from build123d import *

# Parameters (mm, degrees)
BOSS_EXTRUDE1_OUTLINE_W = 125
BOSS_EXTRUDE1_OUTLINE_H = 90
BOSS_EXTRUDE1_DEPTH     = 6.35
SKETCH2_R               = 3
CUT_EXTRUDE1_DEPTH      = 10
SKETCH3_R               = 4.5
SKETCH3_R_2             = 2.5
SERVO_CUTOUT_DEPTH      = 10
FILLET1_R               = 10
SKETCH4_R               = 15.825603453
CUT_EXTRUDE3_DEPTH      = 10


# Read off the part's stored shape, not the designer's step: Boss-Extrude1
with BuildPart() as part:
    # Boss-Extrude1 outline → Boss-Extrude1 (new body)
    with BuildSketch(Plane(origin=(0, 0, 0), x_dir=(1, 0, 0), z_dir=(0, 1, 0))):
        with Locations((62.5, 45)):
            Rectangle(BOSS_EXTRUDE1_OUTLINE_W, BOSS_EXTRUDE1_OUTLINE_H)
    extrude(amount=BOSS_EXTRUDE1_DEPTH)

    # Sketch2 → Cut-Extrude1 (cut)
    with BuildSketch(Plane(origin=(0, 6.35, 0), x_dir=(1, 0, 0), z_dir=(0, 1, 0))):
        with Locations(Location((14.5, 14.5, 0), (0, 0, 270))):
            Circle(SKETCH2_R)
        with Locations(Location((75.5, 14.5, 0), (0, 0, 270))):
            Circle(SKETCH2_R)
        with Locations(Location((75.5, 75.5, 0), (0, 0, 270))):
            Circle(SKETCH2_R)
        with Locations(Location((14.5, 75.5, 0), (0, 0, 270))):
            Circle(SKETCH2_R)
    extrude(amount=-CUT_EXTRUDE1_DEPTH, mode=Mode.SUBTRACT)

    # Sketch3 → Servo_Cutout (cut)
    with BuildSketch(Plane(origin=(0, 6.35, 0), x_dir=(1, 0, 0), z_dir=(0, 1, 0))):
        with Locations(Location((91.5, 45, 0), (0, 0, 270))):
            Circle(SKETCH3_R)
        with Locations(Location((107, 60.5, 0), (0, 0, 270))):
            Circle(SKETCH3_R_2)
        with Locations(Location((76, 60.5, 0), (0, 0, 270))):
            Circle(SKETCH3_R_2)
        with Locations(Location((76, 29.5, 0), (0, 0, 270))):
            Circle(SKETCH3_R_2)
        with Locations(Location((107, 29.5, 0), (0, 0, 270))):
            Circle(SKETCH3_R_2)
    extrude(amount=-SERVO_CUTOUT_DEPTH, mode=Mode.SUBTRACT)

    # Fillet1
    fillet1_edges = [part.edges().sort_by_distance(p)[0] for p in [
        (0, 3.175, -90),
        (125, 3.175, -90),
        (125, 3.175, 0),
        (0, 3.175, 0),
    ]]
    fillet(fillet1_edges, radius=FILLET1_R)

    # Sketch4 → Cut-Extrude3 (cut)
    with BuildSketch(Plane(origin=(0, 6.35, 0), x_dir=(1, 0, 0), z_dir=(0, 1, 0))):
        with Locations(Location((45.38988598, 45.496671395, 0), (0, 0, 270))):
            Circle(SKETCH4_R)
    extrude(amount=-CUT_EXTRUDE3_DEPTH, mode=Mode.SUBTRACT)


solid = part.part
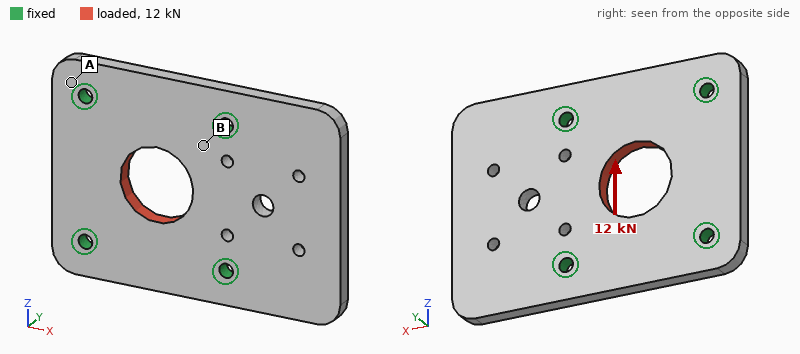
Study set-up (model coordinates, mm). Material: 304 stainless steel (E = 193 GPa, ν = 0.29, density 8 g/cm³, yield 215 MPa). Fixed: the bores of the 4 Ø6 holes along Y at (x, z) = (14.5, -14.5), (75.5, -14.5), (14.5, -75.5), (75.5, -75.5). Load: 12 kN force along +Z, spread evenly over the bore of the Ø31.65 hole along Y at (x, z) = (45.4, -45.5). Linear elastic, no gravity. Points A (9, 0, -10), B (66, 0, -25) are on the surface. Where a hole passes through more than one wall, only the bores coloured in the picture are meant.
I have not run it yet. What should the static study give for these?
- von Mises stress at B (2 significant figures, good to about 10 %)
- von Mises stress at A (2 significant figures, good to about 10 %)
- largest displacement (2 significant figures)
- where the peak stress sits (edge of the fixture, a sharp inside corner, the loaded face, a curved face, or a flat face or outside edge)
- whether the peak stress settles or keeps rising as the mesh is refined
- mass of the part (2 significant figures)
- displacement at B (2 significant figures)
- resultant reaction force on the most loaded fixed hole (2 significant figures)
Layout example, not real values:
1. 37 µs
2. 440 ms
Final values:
1. 21 MPa
2. 9.8 MPa
3. 5.2 µm
4. edge of the fixture
5. keeps rising
6. 510 g
7. 2.3 µm
8. 3.2 kN
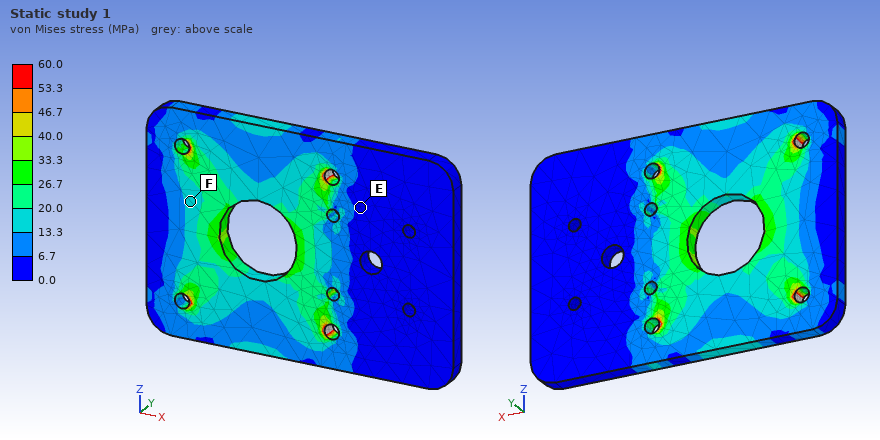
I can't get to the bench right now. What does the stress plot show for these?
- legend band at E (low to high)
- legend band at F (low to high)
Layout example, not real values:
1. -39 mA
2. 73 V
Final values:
1. 0.0 to 6.7 MPa
2. 13.3 to 20.0 MPa
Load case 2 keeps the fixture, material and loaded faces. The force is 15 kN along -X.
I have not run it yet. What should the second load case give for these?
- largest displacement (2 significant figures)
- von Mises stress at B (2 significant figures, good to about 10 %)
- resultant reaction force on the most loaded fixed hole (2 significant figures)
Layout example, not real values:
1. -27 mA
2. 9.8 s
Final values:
1. 6.6 µm
2. 26 MPa
3. 4.0 kN
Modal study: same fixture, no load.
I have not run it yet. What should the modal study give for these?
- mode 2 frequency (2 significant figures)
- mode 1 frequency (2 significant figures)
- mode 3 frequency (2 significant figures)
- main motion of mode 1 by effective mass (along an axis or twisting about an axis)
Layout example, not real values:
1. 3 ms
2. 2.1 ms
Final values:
1. 3300 Hz
2. 1800 Hz
3. 5900 Hz
4. along Y
